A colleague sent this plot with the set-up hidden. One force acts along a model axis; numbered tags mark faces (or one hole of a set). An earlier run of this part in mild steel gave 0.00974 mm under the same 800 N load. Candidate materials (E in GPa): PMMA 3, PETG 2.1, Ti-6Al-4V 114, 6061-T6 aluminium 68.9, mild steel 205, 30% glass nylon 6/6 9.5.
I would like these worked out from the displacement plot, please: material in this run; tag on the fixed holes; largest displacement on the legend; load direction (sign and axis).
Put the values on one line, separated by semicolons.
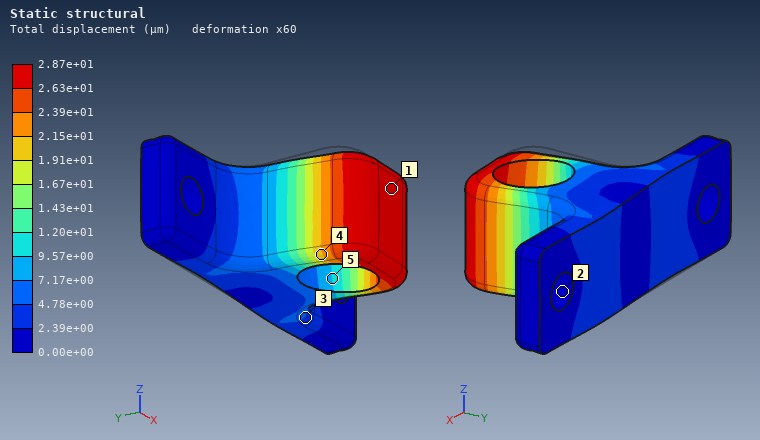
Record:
6061-T6 aluminium; 2; 2.87e+01 µm; +X
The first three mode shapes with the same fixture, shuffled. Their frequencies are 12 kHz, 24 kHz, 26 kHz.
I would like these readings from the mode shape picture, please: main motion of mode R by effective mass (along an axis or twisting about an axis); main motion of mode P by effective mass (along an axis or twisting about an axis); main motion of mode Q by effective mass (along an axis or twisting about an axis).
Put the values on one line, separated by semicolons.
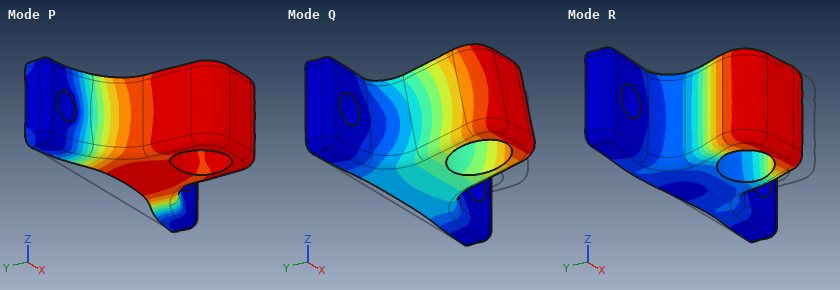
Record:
along X; along Y; along Z
